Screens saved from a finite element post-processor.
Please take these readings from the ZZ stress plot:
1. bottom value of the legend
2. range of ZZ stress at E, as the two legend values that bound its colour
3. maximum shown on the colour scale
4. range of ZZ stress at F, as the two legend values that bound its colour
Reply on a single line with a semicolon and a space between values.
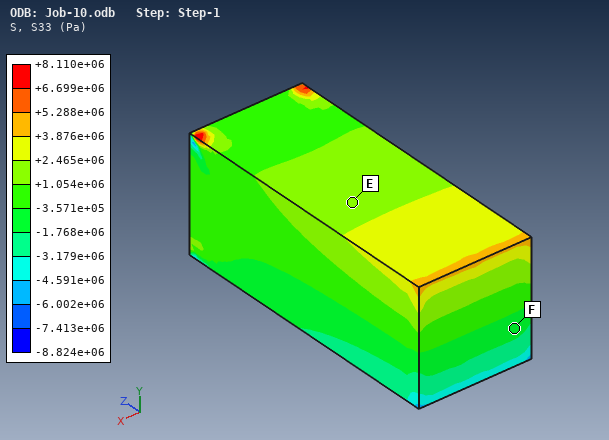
-8.824e+06 Pa; +1.054e+06 to +2.465e+06 Pa; +8.110e+06 Pa; -1.768e+06 to -3.571e+05 Pa
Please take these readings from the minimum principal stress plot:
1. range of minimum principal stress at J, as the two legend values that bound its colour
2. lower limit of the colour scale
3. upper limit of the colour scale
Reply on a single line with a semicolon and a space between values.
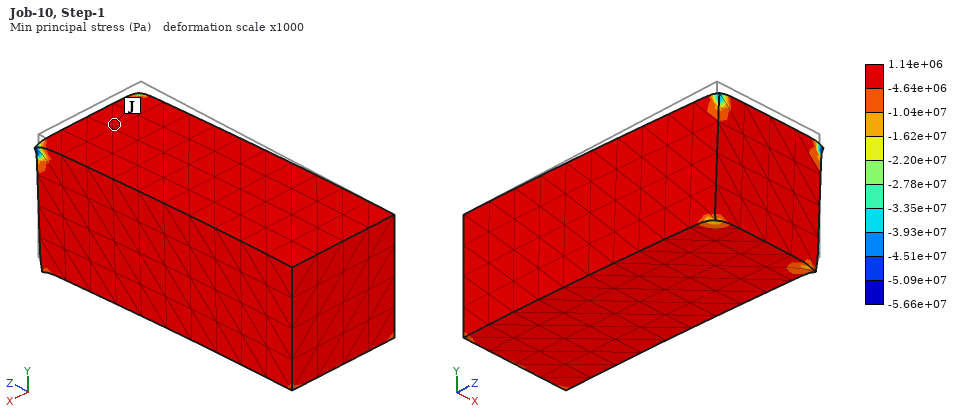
-4.64e+06 to 1.14e+06 Pa; -5.66e+07 Pa; 1.14e+06 Pa
